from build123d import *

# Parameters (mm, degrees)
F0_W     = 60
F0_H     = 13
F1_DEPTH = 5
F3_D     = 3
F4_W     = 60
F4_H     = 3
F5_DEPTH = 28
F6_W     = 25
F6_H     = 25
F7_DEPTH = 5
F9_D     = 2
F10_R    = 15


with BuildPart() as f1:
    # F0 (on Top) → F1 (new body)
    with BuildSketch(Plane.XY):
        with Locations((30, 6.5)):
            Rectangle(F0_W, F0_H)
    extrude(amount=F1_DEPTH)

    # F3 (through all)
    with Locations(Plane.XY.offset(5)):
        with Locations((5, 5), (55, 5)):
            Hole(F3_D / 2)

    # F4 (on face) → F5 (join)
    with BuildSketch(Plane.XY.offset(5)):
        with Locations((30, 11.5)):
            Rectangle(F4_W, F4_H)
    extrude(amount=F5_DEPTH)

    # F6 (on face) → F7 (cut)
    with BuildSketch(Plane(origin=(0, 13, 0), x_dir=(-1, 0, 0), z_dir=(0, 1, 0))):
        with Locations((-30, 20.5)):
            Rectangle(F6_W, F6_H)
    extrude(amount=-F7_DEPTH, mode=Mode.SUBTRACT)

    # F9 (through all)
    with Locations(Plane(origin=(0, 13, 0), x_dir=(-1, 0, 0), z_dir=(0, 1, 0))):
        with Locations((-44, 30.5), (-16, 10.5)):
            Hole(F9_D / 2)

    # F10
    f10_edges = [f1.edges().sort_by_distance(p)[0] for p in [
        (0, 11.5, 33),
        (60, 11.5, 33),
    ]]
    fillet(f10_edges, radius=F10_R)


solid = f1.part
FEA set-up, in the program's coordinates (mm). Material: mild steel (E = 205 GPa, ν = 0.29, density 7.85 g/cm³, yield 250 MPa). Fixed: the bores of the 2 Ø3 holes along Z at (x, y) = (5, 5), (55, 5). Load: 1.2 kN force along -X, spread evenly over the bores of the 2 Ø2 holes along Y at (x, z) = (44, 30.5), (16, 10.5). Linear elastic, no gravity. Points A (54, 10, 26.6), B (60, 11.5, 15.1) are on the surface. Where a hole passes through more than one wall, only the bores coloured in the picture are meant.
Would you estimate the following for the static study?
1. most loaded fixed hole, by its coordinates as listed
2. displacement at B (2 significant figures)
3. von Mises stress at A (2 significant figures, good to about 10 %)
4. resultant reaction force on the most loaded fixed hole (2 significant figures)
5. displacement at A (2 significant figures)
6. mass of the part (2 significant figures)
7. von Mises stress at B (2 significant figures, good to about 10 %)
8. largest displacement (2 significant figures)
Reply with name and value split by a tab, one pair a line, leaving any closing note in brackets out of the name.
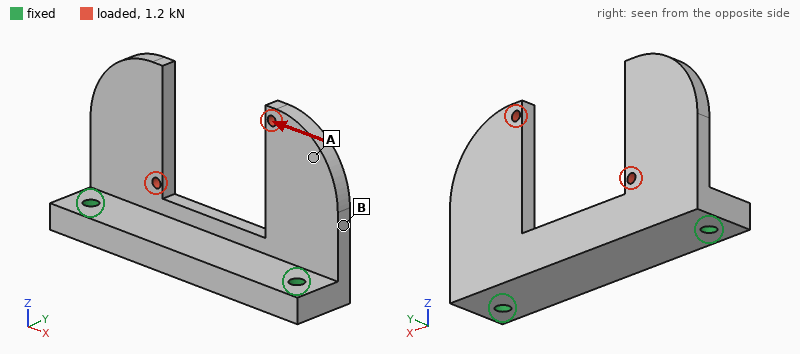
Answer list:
most loaded fixed hole, by its coordinates as listed	(5, 5)
displacement at B	23 µm
von Mises stress at A	30 MPa
resultant reaction force on the most loaded fixed hole	800 N
displacement at A	42 µm
mass of the part	52 g
von Mises stress at B	59 MPa
largest displacement	60 µm
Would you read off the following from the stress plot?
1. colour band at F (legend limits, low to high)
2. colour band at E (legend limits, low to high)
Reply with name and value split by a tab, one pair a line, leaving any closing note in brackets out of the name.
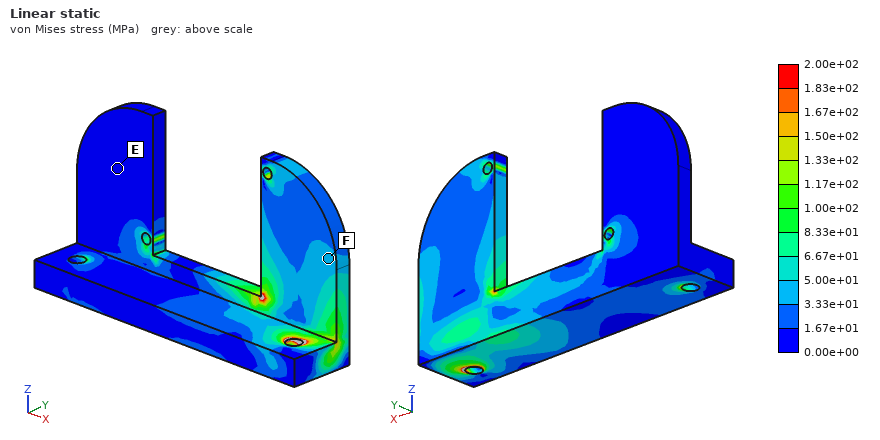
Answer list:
colour band at F	3.33e+01 to 5.00e+01 MPa
colour band at E	0.00e+00 to 1.67e+01 MPa
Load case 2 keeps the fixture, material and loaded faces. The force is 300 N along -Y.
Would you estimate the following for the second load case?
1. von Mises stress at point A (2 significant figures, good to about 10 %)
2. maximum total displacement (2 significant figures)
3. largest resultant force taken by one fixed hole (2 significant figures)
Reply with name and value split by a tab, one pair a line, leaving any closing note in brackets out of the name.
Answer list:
von Mises stress at point A	45 MPa
maximum total displacement	0.18 mm
largest resultant force taken by one fixed hole	170 N
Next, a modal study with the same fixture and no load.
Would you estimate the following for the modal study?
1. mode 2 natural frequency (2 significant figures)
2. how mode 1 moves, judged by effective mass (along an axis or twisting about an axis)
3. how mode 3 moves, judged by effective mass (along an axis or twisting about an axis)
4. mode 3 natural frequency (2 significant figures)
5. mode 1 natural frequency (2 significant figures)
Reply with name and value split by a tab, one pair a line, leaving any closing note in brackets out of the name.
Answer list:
mode 2 natural frequency	3200 Hz
how mode 1 moves, judged by effective mass	along Y
how mode 3 moves, judged by effective mass	along Z
mode 3 natural frequency	6400 Hz
mode 1 natural frequency	3000 Hz
